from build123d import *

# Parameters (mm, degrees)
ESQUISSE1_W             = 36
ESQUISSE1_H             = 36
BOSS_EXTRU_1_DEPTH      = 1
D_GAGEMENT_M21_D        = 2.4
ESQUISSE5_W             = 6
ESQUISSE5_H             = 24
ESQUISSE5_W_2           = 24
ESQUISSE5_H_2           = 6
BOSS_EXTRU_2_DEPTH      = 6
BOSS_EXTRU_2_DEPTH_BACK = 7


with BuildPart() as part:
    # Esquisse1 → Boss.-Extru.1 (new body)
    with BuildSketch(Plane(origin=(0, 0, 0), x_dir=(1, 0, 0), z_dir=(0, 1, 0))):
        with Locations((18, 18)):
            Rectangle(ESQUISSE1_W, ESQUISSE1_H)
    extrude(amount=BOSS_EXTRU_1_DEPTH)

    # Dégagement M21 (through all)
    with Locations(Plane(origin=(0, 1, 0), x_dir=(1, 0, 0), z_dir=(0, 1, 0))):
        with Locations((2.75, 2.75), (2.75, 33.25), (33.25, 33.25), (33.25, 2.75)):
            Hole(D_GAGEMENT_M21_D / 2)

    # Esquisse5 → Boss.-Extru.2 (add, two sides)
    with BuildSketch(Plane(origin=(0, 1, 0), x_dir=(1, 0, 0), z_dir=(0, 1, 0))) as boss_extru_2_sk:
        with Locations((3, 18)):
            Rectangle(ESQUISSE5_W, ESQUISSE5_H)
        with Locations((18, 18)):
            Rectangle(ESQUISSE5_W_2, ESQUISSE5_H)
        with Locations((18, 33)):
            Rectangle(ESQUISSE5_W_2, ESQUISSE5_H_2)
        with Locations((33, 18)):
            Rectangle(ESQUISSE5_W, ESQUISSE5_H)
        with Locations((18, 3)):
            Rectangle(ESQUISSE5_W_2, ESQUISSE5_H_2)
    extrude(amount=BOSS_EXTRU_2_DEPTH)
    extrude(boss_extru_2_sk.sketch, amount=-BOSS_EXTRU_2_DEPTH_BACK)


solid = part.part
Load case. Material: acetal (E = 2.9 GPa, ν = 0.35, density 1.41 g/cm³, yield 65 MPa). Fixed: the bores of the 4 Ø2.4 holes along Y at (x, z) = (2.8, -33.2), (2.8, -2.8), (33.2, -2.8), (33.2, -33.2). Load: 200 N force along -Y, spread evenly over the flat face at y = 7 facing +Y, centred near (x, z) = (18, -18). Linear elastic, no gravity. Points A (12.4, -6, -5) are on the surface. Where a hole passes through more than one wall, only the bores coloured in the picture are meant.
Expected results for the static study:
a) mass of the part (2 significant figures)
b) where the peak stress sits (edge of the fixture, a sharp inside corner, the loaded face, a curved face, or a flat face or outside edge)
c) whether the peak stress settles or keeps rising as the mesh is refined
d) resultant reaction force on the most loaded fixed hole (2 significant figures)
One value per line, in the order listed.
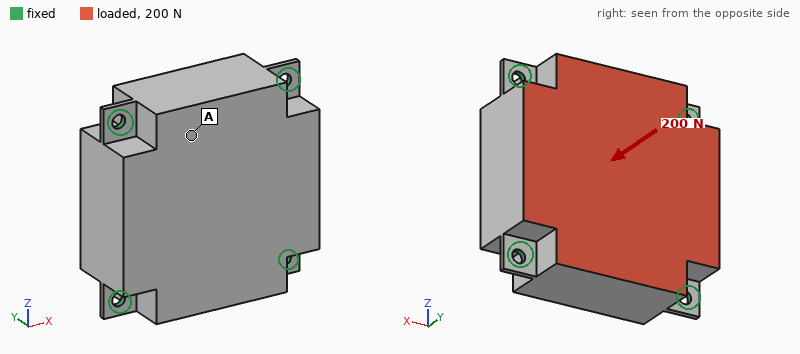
21 g
edge of the fixture
keeps rising
50 N
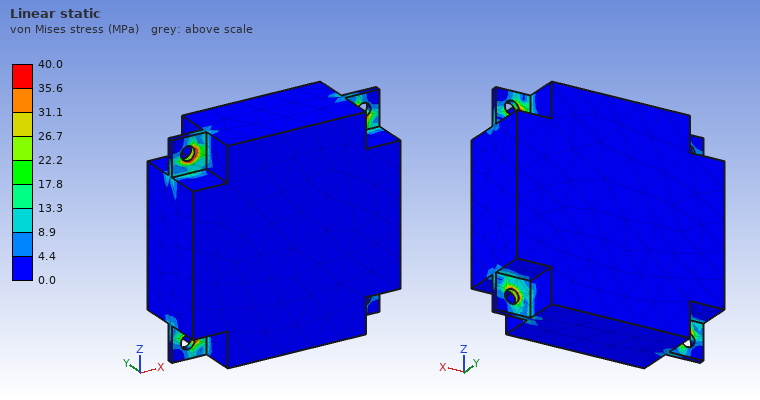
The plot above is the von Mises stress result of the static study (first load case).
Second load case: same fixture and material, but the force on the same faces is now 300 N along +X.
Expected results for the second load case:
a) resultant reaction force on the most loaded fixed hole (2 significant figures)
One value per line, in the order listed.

83 N
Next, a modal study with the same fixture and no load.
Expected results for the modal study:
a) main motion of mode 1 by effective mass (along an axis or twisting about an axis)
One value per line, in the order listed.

along Y
